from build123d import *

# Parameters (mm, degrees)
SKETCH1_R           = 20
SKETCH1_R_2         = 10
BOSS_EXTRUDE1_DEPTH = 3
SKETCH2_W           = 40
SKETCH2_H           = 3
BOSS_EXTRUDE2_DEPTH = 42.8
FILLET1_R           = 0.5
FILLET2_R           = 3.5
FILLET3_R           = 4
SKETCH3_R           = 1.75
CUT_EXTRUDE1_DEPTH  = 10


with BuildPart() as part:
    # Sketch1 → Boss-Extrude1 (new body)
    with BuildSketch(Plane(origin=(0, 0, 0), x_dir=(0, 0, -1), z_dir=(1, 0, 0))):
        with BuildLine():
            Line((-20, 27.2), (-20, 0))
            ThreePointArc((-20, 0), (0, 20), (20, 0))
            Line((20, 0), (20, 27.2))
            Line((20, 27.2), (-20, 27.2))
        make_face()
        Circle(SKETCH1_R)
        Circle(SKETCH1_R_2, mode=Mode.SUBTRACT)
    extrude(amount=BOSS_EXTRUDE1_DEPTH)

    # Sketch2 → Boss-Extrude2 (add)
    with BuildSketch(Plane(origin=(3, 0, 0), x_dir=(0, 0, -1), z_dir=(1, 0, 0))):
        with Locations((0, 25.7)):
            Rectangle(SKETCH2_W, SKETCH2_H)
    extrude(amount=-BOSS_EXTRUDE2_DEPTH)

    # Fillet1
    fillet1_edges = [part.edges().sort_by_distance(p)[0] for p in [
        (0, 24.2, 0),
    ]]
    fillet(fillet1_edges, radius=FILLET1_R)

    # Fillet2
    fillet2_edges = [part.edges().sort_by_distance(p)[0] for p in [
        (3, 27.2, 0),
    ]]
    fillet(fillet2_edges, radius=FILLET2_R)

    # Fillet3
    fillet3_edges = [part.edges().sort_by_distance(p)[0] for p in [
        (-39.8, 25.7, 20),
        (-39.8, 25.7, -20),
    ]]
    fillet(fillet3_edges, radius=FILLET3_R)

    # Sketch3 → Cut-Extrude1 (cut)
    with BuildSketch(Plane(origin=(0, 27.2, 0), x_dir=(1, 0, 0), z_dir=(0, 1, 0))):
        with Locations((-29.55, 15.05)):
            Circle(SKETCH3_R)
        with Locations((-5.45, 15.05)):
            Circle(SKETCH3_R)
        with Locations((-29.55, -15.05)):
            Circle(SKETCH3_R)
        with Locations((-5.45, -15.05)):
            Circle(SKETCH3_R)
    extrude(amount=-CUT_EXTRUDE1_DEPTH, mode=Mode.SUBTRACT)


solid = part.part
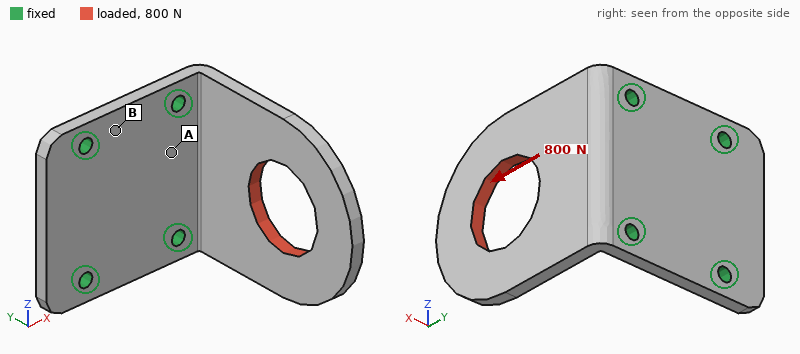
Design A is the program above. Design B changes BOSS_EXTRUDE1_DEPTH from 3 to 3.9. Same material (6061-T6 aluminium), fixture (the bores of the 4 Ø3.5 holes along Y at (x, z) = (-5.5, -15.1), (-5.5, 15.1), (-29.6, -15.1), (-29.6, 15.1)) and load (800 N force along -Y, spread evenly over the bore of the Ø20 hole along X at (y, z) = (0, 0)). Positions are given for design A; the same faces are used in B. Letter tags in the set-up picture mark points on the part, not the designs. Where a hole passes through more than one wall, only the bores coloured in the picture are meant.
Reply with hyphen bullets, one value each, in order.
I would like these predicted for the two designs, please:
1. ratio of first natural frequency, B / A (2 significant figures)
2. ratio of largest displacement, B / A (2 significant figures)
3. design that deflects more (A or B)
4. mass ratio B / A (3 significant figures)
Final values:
- 1.1
- 1.1
- B
- 1.14
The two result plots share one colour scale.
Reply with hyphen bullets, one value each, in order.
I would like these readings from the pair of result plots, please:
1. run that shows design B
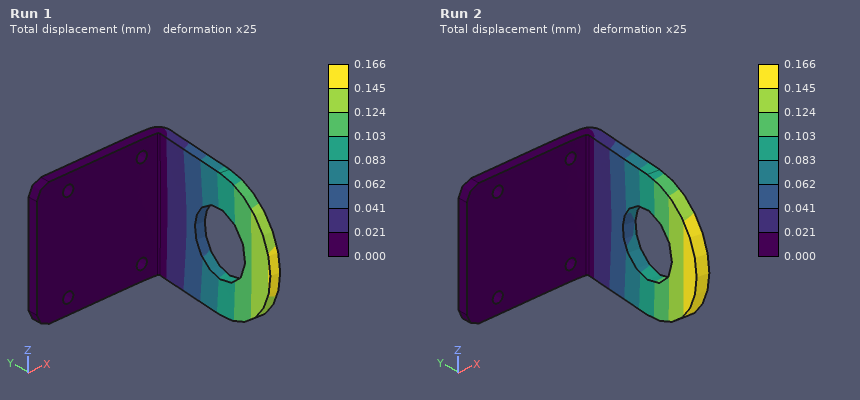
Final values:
- Run 2
